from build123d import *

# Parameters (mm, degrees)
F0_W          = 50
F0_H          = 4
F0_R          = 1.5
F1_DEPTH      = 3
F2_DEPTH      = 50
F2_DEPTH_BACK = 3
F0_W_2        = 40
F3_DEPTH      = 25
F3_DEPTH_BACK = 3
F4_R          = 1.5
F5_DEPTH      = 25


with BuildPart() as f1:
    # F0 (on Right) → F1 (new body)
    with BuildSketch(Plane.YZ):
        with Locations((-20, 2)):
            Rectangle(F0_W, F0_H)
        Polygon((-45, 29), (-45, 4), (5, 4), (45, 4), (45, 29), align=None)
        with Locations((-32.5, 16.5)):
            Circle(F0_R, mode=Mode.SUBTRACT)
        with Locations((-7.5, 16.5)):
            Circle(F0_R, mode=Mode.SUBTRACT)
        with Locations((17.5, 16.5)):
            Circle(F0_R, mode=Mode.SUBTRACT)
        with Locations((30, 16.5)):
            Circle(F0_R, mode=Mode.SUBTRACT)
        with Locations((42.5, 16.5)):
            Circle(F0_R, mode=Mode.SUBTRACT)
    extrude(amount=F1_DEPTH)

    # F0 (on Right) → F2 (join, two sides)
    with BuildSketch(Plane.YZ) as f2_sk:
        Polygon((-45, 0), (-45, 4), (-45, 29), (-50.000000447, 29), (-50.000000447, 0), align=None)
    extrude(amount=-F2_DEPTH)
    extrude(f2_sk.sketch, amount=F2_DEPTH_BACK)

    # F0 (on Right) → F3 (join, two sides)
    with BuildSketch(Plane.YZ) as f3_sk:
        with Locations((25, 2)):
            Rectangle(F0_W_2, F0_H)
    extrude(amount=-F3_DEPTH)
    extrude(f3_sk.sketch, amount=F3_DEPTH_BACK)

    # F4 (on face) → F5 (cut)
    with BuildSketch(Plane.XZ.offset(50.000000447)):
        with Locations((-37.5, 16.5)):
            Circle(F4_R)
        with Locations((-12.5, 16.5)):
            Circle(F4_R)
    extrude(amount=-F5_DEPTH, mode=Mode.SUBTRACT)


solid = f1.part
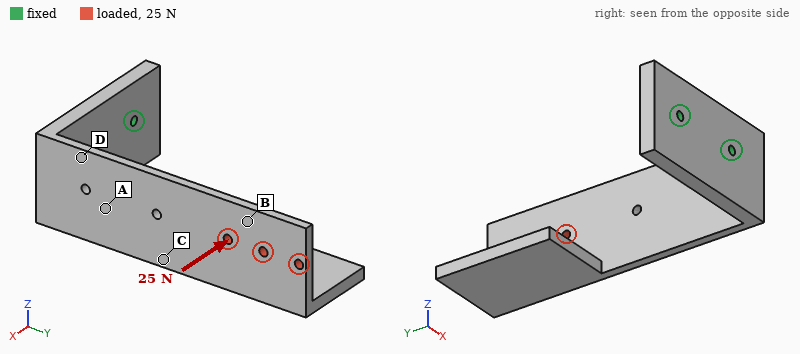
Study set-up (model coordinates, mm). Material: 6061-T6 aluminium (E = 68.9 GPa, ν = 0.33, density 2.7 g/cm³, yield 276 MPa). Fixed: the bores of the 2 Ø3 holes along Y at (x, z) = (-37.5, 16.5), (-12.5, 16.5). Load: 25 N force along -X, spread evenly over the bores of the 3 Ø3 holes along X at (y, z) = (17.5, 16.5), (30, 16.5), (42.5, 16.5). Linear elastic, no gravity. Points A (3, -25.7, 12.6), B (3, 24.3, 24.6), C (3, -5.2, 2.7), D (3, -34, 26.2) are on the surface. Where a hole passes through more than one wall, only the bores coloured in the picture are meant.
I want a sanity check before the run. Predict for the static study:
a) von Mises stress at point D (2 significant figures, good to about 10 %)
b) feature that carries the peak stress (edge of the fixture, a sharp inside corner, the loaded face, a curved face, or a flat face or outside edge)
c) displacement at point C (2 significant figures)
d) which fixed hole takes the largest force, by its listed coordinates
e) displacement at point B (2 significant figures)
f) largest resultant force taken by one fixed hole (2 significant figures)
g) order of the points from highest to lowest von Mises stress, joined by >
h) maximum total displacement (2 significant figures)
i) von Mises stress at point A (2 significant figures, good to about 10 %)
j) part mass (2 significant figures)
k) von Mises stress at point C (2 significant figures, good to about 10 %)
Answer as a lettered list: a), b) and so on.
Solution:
a) 39 MPa
b) a curved face
c) 0.34 mm
d) (-12.5, 16.5)
e) 0.81 mm
f) 44 N
g) D > A > C > B
h) 1.2 mm
i) 30 MPa
j) 52 g
k) 22 MPa
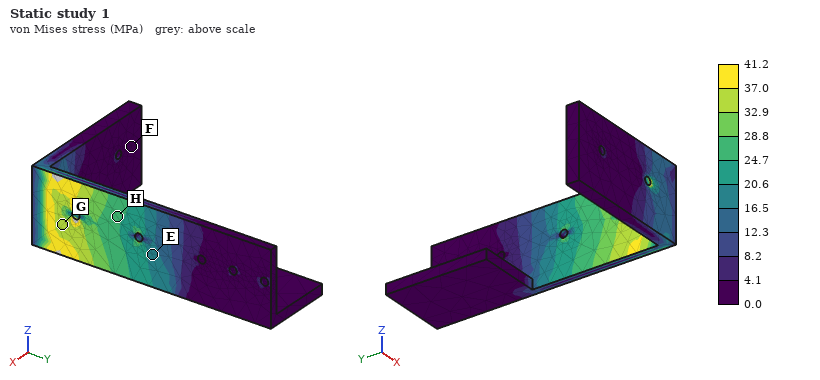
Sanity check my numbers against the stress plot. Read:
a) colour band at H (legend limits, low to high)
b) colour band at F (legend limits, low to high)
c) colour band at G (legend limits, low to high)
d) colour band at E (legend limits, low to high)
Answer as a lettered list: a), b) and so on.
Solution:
a) 24.7 to 28.8 MPa
b) 0.0 to 4.1 MPa
c) 32.9 to 37.0 MPa
d) 16.5 to 20.6 MPa
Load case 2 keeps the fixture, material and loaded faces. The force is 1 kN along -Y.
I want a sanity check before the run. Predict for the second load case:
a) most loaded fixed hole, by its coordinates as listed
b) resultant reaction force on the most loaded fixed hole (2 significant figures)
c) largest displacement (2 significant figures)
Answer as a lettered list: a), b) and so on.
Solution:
a) (-12.5, 16.5)
b) 1.2 kN
c) 0.57 mm
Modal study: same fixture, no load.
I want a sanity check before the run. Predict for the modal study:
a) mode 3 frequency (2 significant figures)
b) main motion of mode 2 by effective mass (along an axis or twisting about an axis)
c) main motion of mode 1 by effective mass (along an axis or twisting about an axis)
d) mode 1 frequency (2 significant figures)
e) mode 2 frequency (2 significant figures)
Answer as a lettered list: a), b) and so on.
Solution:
a) 1000 Hz
b) along Z
c) along X
d) 190 Hz
e) 510 Hz
